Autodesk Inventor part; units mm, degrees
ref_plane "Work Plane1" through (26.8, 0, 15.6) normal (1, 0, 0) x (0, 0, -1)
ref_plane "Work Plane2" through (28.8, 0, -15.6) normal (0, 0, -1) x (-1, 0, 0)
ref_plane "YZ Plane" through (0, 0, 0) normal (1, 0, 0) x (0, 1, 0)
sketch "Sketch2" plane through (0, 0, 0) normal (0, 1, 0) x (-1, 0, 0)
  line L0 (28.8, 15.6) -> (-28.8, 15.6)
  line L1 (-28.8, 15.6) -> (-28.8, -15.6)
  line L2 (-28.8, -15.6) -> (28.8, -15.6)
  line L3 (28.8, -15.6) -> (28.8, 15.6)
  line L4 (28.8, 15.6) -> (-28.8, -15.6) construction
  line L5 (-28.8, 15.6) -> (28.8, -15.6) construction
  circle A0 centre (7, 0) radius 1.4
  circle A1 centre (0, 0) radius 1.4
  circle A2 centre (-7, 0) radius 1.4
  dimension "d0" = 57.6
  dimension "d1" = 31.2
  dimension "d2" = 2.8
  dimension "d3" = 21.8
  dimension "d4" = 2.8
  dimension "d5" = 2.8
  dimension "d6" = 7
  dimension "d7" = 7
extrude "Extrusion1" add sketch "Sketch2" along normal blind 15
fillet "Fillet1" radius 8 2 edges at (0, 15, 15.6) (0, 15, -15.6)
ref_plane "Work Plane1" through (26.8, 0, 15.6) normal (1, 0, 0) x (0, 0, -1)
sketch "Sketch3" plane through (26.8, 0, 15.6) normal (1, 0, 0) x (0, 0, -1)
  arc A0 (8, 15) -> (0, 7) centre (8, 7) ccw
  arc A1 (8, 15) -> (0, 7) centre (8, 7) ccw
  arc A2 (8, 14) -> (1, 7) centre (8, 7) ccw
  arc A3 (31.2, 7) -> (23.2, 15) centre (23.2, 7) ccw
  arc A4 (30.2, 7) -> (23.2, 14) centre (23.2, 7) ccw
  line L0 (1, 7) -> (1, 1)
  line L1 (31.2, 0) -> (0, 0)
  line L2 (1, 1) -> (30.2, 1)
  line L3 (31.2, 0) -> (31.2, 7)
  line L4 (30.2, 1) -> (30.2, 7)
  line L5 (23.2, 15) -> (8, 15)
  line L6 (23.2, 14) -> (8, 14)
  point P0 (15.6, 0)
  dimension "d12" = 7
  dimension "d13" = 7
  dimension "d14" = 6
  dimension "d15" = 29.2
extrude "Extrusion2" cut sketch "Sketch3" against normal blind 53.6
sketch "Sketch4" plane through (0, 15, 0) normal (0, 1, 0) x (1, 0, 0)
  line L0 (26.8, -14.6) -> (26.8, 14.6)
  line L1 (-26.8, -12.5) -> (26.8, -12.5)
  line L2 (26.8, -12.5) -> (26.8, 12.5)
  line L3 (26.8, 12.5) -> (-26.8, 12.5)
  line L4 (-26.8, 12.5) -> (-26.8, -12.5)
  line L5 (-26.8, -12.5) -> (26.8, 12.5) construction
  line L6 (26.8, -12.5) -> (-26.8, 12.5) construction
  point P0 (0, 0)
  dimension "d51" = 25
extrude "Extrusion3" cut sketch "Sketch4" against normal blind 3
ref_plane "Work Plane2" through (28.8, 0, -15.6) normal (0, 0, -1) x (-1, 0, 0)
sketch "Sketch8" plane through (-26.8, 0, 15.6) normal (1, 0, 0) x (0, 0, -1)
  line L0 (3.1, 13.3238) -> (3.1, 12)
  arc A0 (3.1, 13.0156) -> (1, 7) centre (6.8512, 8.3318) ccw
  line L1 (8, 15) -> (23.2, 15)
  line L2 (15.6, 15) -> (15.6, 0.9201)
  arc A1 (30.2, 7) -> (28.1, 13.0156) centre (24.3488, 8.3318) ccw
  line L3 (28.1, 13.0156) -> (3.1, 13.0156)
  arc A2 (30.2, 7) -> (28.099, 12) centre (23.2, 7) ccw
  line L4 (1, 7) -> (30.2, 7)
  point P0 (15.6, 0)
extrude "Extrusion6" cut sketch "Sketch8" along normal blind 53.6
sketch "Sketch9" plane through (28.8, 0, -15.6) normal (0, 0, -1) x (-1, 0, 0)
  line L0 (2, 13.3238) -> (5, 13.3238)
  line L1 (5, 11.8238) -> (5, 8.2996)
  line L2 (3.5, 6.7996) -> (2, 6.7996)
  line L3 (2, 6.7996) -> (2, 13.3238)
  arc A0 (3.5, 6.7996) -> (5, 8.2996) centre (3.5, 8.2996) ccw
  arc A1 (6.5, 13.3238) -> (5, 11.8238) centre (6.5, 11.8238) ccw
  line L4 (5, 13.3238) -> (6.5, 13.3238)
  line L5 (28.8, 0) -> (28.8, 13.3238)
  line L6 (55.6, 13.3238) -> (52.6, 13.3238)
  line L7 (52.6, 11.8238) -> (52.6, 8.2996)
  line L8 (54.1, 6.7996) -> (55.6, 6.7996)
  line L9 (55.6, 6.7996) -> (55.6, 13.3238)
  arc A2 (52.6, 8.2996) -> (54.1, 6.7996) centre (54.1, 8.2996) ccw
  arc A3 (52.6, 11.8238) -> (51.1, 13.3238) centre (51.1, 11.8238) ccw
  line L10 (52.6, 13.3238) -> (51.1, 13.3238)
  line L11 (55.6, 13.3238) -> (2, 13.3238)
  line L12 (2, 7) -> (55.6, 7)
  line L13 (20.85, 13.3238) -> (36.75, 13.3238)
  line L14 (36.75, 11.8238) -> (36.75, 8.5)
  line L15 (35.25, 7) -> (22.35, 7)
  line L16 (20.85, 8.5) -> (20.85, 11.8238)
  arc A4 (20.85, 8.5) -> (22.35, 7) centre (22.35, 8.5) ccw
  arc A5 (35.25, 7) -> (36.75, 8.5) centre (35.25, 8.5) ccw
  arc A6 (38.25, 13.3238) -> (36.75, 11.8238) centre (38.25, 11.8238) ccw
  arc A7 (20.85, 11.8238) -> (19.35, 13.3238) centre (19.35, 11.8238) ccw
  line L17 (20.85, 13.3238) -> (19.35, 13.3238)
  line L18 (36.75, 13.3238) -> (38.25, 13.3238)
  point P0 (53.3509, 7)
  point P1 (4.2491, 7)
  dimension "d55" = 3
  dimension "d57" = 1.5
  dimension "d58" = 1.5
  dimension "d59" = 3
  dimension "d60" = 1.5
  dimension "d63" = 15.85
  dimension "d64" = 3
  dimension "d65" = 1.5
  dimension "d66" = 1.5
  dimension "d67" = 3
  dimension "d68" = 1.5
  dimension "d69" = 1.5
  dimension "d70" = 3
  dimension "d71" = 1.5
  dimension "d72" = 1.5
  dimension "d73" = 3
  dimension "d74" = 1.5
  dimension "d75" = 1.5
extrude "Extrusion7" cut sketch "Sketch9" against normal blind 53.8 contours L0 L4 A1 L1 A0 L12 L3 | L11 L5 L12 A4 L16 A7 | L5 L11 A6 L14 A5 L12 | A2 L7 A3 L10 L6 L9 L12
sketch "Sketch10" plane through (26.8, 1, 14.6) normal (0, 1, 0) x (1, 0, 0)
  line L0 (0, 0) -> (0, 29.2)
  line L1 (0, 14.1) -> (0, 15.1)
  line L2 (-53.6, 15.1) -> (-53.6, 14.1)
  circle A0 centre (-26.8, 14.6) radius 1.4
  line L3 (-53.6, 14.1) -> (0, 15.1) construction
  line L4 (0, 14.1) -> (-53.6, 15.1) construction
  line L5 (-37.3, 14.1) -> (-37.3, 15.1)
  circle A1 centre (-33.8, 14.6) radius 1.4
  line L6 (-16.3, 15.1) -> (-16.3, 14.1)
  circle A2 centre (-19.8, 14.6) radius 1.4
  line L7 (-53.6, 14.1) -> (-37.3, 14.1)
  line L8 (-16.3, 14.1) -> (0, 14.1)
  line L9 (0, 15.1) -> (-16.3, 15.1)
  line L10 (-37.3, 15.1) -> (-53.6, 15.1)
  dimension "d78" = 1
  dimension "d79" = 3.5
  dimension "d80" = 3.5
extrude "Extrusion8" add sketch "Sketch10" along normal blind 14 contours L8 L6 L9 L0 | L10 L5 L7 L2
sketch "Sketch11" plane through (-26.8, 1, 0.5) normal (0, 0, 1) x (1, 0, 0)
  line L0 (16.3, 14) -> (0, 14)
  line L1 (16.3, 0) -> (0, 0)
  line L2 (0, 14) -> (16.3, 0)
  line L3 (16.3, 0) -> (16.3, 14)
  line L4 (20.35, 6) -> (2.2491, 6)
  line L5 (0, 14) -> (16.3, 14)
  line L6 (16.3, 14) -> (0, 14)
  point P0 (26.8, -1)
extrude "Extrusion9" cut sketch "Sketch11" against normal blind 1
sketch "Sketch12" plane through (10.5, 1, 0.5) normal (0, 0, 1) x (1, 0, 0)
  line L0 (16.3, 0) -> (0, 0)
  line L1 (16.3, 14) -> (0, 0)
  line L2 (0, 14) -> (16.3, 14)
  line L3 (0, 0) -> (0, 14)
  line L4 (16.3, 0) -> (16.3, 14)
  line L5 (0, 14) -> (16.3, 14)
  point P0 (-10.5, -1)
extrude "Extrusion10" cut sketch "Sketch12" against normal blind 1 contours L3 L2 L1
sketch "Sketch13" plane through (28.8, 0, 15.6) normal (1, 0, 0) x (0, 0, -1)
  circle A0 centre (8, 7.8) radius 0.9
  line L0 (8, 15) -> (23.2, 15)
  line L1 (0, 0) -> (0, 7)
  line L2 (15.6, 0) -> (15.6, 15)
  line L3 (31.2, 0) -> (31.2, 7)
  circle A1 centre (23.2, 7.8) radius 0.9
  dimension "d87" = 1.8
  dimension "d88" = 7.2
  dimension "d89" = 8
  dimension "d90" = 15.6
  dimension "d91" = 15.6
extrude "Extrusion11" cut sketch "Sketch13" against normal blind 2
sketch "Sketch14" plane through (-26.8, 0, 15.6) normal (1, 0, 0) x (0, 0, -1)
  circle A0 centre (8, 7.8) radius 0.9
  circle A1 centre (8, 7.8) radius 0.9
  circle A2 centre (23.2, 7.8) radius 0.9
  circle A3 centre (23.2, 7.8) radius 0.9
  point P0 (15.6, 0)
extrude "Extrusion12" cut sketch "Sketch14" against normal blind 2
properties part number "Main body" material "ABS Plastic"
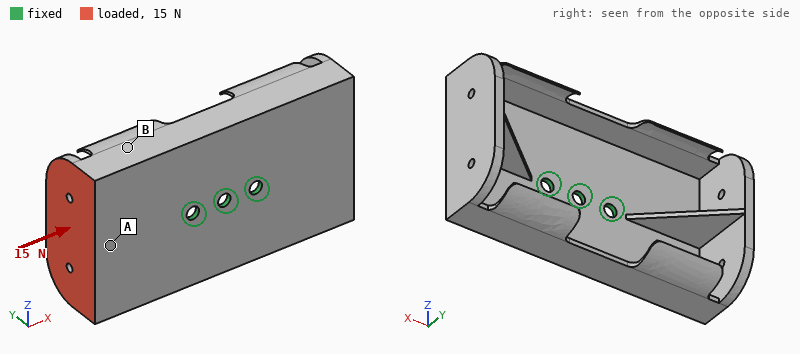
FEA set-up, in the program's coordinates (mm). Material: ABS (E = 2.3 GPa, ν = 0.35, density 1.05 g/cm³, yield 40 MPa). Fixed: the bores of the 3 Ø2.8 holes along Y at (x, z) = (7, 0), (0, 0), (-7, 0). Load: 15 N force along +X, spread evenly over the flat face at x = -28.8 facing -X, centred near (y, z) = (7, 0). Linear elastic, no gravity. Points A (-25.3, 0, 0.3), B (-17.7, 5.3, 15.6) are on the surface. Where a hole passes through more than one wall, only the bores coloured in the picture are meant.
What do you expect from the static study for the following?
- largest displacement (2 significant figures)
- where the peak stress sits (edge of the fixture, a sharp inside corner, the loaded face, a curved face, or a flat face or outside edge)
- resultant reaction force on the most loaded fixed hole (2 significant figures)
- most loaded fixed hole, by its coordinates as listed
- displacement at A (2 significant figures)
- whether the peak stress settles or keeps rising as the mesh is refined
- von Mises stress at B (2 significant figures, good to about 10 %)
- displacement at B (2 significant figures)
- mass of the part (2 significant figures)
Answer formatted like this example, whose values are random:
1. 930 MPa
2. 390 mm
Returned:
1. 0.74 mm
2. edge of the fixture
3. 8.3 N
4. (-7, 0)
5. 0.48 mm
6. keeps rising
7. 1.9 MPa
8. 0.37 mm
9. 4.7 g
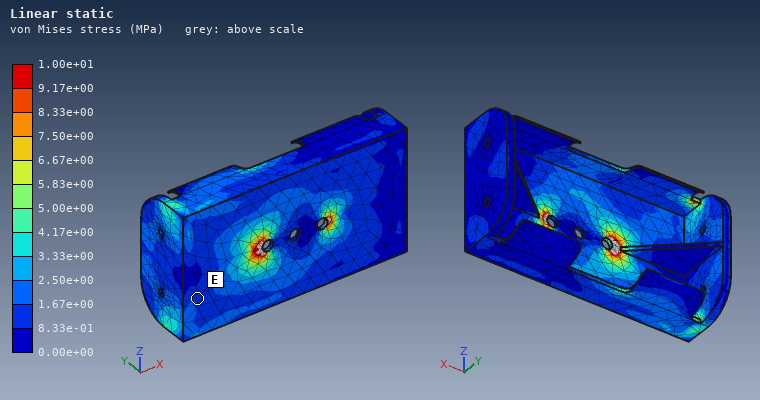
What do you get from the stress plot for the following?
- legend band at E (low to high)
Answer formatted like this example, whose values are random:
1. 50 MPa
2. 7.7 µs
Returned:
1. 8.33e-01 to 1.67e+00 MPa
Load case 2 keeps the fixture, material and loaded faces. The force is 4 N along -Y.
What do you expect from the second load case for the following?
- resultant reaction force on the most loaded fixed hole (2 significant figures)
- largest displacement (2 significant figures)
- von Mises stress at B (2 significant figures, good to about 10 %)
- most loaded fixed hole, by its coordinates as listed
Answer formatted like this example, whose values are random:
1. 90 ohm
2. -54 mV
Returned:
1. 7.9 N
2. 0.65 mm
3. 1.4 MPa
4. (-7, 0)
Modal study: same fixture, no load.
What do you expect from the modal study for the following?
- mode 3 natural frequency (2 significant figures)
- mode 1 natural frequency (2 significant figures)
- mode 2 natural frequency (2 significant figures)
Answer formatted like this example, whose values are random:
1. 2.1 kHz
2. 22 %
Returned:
1. 460 Hz
2. 300 Hz
3. 350 Hz
